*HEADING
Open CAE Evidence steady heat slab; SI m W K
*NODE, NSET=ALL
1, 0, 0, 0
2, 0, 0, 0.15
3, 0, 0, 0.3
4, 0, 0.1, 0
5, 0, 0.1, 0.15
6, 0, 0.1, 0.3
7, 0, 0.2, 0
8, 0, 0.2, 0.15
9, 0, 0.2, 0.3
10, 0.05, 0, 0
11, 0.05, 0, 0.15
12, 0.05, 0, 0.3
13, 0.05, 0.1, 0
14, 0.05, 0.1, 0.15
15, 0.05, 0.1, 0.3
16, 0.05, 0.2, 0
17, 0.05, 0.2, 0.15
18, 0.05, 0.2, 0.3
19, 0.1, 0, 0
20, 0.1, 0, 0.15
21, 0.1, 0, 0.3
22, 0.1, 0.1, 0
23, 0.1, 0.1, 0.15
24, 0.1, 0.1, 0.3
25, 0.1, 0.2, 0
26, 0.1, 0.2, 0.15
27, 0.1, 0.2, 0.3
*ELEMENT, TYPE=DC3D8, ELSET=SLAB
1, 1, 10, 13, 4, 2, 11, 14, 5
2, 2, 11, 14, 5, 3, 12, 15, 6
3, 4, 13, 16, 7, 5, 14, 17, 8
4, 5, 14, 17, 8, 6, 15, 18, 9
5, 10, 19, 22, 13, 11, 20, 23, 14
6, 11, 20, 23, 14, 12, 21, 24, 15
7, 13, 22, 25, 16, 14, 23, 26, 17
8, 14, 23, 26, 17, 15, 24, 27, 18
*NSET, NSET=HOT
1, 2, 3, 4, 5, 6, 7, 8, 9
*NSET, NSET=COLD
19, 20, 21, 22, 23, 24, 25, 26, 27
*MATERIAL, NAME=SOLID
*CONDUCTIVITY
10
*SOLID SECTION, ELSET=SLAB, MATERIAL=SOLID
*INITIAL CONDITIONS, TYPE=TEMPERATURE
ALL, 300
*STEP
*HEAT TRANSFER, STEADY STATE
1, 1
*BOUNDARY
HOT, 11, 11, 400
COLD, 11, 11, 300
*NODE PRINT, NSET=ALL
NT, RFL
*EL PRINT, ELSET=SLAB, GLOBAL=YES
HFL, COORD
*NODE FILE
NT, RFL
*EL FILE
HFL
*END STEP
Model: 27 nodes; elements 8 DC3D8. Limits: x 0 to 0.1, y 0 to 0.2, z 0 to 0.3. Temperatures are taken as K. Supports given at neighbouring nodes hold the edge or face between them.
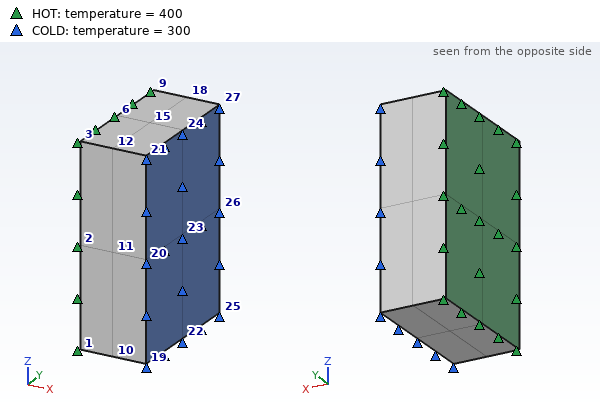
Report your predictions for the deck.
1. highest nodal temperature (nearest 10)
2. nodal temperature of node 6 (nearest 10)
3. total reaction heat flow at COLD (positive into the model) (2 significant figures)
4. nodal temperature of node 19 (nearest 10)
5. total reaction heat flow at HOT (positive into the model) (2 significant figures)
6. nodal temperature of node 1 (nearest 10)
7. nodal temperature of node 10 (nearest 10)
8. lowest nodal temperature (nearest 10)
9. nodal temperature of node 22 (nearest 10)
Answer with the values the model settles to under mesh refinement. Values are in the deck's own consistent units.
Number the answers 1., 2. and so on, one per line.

1. 400 K
2. 400 K
3. -600
4. 300 K
5. 600
6. 400 K
7. 350 K
8. 300 K
9. 300 K
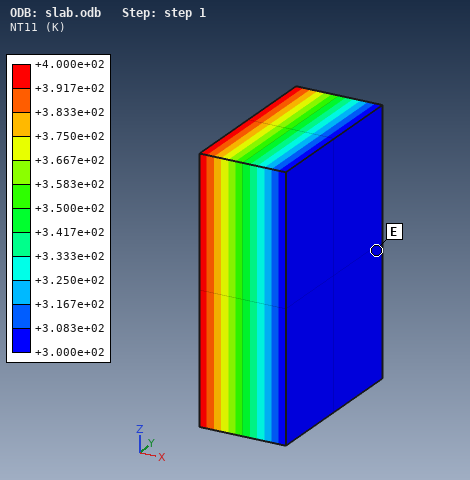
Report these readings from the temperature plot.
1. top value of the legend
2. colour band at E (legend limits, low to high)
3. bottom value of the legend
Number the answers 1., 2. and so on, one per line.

1. +4.000e+02 K
2. +3.000e+02 to +3.083e+02 K
3. +3.000e+02 K
